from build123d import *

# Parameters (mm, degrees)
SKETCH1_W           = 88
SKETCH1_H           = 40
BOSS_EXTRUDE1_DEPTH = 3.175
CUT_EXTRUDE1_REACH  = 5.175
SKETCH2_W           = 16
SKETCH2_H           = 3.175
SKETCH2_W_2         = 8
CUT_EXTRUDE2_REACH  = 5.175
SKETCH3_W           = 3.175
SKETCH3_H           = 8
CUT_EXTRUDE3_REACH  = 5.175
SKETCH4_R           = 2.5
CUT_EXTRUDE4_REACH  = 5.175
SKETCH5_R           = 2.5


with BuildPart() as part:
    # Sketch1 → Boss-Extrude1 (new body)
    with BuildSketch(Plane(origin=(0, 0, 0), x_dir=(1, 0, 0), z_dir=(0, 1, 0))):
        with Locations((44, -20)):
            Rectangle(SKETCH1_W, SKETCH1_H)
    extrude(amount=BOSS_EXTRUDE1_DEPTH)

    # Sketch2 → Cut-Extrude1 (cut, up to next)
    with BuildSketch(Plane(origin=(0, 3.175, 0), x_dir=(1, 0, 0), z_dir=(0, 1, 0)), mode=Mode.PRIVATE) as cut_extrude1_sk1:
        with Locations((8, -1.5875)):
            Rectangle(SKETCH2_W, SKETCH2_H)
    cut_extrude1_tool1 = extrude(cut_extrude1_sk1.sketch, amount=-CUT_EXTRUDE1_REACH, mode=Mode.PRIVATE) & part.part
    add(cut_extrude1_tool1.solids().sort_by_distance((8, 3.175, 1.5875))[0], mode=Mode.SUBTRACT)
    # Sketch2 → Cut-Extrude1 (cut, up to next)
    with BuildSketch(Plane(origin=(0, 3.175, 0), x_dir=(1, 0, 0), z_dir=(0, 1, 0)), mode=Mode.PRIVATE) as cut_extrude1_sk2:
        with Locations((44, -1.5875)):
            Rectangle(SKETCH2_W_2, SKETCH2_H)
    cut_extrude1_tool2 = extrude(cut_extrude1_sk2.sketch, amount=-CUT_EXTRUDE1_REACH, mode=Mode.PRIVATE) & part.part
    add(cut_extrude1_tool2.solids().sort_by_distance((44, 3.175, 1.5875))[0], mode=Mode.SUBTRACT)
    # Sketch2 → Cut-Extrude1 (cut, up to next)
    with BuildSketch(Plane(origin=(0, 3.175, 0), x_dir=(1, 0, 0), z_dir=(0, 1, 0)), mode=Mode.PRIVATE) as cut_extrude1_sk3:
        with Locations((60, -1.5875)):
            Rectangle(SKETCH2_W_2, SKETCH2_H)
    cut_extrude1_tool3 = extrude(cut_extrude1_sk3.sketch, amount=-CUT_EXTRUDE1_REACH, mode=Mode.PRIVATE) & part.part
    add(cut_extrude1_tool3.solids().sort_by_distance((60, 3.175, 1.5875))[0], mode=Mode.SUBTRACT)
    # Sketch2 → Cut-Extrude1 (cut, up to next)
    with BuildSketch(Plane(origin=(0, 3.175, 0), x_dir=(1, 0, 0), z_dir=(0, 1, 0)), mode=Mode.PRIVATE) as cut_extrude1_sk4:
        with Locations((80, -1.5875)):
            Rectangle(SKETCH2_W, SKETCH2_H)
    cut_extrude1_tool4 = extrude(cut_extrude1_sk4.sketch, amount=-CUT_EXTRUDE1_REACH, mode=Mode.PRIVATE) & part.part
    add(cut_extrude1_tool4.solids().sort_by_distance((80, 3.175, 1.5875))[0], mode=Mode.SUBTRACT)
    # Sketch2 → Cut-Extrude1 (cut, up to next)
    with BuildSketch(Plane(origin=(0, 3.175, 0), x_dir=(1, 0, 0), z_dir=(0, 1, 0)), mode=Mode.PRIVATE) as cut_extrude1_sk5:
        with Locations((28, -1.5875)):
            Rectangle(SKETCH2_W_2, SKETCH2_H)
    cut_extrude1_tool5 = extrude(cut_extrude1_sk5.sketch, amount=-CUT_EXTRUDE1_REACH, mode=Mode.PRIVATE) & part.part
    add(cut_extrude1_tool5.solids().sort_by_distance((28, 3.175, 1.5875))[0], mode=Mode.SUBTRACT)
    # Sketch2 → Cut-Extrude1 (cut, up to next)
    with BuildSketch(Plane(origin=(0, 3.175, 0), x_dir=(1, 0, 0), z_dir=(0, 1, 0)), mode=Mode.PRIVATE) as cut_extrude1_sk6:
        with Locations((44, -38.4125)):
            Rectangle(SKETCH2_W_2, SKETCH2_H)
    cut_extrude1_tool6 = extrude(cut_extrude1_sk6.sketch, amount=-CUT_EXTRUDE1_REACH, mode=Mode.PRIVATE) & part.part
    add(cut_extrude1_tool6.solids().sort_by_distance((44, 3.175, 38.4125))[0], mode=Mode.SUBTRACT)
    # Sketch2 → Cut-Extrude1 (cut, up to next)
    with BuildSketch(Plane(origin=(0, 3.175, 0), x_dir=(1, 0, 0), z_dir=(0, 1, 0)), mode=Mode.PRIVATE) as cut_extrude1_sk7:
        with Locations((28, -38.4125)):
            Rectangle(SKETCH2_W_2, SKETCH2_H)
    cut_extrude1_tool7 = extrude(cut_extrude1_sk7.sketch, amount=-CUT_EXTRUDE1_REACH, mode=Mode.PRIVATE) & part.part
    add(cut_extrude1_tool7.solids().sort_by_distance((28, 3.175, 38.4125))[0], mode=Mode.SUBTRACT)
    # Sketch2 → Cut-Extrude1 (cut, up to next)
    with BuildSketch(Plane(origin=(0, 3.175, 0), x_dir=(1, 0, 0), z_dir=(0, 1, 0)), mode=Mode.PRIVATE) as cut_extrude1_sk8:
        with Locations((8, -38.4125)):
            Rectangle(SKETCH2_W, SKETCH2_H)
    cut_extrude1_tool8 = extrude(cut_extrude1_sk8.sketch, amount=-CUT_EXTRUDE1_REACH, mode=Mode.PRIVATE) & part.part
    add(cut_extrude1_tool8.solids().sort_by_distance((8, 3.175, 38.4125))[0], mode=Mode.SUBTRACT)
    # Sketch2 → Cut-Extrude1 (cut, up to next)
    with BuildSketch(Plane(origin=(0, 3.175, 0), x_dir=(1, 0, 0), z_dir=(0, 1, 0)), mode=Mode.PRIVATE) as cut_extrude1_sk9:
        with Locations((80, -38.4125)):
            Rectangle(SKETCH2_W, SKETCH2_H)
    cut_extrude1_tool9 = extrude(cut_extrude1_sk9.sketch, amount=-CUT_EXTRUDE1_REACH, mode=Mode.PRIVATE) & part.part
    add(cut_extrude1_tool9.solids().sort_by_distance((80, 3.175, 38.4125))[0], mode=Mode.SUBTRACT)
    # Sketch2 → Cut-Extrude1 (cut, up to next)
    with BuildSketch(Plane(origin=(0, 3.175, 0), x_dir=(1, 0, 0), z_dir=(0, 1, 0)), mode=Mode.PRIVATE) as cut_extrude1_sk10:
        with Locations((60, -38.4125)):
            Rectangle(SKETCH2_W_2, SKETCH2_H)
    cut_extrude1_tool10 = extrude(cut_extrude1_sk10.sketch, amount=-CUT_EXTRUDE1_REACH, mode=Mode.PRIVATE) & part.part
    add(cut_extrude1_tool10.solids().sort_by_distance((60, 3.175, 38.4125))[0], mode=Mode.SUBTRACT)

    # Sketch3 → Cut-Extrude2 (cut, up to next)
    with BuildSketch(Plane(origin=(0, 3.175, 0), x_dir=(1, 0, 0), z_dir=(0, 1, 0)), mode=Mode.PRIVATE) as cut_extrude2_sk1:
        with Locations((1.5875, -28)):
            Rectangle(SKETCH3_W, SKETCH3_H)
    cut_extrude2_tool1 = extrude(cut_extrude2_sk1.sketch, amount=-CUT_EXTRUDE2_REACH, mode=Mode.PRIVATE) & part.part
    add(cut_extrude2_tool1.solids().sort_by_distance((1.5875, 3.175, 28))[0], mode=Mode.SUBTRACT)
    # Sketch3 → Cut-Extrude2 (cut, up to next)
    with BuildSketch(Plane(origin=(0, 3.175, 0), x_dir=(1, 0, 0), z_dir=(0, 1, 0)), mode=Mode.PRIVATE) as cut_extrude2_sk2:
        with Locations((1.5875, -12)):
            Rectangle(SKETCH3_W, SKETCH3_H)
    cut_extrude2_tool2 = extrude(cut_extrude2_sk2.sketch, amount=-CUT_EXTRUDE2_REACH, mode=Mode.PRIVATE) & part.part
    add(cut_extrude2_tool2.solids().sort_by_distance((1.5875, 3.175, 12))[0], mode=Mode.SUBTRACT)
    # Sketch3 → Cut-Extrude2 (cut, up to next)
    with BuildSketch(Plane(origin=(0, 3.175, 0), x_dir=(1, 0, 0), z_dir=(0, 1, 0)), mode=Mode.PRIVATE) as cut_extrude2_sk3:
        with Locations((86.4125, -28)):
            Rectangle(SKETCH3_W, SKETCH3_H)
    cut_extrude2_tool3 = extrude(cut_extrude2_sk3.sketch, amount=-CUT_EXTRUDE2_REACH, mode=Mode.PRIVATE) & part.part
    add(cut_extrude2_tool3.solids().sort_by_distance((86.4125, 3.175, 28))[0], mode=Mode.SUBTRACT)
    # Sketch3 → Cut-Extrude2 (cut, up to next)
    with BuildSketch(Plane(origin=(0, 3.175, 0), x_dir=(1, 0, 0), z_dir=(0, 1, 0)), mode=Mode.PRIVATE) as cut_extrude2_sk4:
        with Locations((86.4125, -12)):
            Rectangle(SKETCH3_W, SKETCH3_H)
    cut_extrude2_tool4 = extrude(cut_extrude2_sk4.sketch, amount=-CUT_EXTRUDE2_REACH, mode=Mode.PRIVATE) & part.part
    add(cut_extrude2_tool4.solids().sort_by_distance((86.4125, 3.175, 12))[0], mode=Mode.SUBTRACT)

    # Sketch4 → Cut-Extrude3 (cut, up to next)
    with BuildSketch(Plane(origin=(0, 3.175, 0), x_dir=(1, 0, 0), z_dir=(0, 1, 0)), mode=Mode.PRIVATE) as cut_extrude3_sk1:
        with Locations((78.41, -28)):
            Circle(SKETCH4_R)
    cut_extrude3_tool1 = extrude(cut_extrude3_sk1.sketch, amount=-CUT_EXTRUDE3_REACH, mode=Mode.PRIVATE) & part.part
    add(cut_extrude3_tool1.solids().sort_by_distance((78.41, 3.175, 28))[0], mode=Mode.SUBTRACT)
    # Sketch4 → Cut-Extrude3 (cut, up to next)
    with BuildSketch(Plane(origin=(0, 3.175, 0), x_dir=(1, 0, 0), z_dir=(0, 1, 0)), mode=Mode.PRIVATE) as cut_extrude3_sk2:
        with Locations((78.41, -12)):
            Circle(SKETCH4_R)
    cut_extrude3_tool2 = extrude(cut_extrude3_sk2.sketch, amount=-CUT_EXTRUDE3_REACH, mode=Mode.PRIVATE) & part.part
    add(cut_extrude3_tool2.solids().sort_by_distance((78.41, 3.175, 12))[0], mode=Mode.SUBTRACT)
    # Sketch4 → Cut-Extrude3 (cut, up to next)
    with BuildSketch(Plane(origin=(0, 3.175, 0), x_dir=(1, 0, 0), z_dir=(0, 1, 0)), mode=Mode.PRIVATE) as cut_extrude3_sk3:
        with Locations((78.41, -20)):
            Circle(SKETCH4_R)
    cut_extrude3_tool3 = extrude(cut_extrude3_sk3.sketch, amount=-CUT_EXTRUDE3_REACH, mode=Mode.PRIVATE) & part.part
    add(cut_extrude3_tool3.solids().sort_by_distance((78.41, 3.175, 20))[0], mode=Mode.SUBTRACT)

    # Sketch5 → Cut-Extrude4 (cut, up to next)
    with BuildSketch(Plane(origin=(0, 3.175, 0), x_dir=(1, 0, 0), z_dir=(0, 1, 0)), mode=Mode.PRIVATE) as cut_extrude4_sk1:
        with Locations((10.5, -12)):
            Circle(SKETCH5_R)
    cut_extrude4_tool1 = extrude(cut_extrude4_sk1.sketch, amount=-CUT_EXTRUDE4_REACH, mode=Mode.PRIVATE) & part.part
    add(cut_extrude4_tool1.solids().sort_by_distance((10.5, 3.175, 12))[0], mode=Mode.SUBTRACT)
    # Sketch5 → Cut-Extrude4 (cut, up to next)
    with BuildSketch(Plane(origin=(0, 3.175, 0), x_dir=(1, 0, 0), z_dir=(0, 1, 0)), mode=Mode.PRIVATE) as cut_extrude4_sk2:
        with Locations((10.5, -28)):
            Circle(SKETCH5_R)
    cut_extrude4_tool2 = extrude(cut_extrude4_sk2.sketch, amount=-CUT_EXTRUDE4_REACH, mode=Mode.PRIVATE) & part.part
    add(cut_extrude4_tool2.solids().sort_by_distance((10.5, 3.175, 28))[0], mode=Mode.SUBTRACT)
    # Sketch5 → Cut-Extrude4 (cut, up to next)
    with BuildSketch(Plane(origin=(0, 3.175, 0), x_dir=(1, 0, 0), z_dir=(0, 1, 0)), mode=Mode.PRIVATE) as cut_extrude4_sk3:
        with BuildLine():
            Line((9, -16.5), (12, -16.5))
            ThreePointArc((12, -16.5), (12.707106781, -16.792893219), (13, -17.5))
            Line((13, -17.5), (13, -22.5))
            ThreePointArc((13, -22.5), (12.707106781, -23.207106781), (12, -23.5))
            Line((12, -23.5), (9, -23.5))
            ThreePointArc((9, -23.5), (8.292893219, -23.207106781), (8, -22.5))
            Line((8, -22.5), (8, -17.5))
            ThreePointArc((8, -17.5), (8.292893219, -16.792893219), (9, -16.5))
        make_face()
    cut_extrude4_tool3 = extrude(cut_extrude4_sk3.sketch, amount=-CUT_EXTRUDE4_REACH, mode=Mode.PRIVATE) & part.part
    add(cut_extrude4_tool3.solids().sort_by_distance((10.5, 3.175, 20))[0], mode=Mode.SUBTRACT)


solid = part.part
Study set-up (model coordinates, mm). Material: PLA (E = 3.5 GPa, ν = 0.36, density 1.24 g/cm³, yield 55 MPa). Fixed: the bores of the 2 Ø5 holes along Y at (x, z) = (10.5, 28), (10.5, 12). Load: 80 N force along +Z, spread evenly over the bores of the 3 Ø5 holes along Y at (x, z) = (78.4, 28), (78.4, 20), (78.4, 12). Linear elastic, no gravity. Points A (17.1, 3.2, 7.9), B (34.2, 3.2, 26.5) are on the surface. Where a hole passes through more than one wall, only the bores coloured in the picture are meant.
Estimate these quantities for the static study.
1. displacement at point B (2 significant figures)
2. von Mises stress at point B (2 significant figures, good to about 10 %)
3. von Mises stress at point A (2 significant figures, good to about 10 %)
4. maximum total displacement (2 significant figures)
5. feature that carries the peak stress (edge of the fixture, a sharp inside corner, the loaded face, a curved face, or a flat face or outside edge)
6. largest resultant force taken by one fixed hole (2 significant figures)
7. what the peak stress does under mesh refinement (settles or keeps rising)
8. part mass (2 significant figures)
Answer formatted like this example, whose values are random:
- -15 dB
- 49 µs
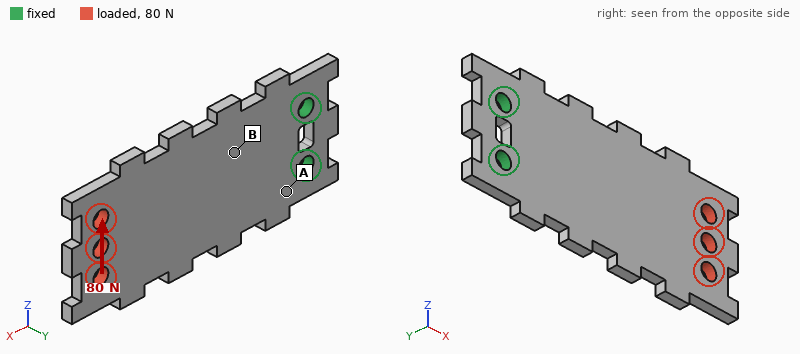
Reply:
- 0.075 mm
- 2.9 MPa
- 5.9 MPa
- 0.40 mm
- edge of the fixture
- 270 N
- keeps rising
- 12 g
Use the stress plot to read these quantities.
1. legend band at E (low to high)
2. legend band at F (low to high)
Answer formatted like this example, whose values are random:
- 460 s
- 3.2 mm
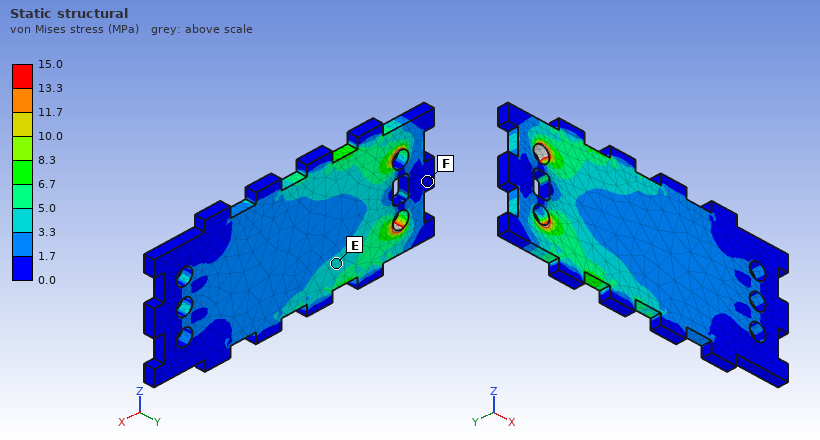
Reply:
- 3.3 to 5.0 MPa
- 0.0 to 1.7 MPa
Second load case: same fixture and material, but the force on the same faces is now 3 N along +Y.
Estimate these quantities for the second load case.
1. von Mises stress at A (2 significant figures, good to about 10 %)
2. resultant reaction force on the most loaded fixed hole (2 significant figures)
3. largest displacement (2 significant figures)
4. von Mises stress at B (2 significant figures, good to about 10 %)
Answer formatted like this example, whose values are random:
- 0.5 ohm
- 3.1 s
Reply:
- 3.0 MPa
- 1.5 N
- 1.1 mm
- 2.1 MPa
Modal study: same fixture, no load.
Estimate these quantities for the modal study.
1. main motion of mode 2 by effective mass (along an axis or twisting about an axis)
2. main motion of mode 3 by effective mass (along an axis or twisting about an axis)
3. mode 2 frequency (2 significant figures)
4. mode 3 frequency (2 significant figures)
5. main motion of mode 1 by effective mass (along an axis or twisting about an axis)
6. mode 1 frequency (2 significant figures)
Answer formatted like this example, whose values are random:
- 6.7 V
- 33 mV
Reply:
- twisting about X
- along Y
- 640 Hz
- 940 Hz
- along Y
- 160 Hz
